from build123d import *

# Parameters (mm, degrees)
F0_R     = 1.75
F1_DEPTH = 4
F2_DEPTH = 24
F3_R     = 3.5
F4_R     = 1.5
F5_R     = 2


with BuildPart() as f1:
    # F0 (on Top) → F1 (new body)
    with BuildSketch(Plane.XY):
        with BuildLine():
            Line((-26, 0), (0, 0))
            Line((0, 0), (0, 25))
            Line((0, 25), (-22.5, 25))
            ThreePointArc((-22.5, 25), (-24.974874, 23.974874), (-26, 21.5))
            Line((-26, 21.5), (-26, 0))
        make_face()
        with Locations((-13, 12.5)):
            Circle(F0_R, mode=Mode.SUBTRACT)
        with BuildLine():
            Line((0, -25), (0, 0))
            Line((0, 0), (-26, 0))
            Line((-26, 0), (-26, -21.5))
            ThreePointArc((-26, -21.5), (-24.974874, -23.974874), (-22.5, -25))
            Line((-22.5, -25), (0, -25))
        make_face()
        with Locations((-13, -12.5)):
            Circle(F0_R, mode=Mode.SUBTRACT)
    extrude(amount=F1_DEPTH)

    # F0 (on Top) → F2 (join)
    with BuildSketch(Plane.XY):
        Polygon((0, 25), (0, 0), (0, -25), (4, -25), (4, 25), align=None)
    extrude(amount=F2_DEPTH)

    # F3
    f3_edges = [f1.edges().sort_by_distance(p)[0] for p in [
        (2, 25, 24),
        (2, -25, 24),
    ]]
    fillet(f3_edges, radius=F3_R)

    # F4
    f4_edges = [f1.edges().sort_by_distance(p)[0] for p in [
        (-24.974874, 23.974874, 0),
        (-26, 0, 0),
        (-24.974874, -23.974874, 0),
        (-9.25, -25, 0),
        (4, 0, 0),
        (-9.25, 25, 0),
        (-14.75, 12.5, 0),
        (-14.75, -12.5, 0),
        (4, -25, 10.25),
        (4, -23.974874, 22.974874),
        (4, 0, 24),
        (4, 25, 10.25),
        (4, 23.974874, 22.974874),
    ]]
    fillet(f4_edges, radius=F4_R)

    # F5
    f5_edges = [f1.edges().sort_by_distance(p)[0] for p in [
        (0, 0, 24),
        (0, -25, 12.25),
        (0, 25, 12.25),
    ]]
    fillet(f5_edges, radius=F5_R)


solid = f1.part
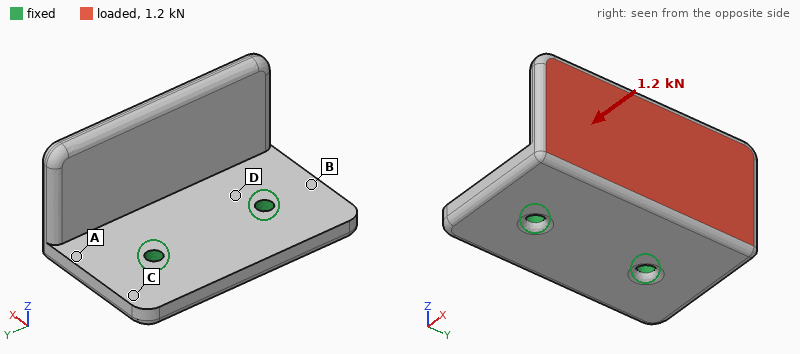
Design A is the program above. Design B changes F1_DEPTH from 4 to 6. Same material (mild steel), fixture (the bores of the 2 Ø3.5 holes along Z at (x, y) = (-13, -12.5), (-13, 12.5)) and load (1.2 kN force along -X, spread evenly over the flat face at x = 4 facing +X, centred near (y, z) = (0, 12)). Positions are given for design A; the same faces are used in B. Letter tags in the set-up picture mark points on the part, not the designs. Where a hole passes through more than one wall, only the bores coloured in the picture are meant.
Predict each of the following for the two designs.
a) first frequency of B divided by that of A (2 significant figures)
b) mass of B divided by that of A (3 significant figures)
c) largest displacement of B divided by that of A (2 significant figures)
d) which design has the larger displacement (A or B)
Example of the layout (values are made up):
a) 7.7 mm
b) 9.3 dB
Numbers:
a) 1.7
b) 1.26
c) 0.35
d) A
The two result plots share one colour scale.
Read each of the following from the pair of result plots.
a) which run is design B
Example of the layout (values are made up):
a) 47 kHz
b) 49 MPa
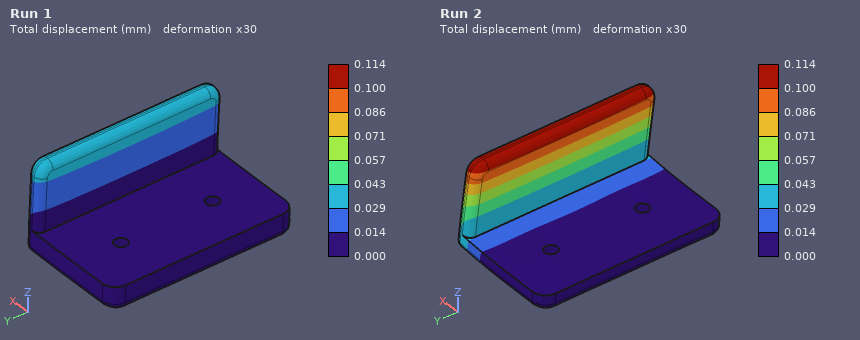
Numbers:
a) Run 1
